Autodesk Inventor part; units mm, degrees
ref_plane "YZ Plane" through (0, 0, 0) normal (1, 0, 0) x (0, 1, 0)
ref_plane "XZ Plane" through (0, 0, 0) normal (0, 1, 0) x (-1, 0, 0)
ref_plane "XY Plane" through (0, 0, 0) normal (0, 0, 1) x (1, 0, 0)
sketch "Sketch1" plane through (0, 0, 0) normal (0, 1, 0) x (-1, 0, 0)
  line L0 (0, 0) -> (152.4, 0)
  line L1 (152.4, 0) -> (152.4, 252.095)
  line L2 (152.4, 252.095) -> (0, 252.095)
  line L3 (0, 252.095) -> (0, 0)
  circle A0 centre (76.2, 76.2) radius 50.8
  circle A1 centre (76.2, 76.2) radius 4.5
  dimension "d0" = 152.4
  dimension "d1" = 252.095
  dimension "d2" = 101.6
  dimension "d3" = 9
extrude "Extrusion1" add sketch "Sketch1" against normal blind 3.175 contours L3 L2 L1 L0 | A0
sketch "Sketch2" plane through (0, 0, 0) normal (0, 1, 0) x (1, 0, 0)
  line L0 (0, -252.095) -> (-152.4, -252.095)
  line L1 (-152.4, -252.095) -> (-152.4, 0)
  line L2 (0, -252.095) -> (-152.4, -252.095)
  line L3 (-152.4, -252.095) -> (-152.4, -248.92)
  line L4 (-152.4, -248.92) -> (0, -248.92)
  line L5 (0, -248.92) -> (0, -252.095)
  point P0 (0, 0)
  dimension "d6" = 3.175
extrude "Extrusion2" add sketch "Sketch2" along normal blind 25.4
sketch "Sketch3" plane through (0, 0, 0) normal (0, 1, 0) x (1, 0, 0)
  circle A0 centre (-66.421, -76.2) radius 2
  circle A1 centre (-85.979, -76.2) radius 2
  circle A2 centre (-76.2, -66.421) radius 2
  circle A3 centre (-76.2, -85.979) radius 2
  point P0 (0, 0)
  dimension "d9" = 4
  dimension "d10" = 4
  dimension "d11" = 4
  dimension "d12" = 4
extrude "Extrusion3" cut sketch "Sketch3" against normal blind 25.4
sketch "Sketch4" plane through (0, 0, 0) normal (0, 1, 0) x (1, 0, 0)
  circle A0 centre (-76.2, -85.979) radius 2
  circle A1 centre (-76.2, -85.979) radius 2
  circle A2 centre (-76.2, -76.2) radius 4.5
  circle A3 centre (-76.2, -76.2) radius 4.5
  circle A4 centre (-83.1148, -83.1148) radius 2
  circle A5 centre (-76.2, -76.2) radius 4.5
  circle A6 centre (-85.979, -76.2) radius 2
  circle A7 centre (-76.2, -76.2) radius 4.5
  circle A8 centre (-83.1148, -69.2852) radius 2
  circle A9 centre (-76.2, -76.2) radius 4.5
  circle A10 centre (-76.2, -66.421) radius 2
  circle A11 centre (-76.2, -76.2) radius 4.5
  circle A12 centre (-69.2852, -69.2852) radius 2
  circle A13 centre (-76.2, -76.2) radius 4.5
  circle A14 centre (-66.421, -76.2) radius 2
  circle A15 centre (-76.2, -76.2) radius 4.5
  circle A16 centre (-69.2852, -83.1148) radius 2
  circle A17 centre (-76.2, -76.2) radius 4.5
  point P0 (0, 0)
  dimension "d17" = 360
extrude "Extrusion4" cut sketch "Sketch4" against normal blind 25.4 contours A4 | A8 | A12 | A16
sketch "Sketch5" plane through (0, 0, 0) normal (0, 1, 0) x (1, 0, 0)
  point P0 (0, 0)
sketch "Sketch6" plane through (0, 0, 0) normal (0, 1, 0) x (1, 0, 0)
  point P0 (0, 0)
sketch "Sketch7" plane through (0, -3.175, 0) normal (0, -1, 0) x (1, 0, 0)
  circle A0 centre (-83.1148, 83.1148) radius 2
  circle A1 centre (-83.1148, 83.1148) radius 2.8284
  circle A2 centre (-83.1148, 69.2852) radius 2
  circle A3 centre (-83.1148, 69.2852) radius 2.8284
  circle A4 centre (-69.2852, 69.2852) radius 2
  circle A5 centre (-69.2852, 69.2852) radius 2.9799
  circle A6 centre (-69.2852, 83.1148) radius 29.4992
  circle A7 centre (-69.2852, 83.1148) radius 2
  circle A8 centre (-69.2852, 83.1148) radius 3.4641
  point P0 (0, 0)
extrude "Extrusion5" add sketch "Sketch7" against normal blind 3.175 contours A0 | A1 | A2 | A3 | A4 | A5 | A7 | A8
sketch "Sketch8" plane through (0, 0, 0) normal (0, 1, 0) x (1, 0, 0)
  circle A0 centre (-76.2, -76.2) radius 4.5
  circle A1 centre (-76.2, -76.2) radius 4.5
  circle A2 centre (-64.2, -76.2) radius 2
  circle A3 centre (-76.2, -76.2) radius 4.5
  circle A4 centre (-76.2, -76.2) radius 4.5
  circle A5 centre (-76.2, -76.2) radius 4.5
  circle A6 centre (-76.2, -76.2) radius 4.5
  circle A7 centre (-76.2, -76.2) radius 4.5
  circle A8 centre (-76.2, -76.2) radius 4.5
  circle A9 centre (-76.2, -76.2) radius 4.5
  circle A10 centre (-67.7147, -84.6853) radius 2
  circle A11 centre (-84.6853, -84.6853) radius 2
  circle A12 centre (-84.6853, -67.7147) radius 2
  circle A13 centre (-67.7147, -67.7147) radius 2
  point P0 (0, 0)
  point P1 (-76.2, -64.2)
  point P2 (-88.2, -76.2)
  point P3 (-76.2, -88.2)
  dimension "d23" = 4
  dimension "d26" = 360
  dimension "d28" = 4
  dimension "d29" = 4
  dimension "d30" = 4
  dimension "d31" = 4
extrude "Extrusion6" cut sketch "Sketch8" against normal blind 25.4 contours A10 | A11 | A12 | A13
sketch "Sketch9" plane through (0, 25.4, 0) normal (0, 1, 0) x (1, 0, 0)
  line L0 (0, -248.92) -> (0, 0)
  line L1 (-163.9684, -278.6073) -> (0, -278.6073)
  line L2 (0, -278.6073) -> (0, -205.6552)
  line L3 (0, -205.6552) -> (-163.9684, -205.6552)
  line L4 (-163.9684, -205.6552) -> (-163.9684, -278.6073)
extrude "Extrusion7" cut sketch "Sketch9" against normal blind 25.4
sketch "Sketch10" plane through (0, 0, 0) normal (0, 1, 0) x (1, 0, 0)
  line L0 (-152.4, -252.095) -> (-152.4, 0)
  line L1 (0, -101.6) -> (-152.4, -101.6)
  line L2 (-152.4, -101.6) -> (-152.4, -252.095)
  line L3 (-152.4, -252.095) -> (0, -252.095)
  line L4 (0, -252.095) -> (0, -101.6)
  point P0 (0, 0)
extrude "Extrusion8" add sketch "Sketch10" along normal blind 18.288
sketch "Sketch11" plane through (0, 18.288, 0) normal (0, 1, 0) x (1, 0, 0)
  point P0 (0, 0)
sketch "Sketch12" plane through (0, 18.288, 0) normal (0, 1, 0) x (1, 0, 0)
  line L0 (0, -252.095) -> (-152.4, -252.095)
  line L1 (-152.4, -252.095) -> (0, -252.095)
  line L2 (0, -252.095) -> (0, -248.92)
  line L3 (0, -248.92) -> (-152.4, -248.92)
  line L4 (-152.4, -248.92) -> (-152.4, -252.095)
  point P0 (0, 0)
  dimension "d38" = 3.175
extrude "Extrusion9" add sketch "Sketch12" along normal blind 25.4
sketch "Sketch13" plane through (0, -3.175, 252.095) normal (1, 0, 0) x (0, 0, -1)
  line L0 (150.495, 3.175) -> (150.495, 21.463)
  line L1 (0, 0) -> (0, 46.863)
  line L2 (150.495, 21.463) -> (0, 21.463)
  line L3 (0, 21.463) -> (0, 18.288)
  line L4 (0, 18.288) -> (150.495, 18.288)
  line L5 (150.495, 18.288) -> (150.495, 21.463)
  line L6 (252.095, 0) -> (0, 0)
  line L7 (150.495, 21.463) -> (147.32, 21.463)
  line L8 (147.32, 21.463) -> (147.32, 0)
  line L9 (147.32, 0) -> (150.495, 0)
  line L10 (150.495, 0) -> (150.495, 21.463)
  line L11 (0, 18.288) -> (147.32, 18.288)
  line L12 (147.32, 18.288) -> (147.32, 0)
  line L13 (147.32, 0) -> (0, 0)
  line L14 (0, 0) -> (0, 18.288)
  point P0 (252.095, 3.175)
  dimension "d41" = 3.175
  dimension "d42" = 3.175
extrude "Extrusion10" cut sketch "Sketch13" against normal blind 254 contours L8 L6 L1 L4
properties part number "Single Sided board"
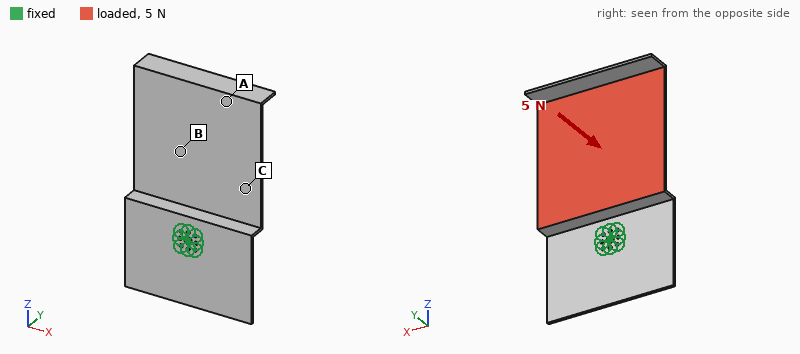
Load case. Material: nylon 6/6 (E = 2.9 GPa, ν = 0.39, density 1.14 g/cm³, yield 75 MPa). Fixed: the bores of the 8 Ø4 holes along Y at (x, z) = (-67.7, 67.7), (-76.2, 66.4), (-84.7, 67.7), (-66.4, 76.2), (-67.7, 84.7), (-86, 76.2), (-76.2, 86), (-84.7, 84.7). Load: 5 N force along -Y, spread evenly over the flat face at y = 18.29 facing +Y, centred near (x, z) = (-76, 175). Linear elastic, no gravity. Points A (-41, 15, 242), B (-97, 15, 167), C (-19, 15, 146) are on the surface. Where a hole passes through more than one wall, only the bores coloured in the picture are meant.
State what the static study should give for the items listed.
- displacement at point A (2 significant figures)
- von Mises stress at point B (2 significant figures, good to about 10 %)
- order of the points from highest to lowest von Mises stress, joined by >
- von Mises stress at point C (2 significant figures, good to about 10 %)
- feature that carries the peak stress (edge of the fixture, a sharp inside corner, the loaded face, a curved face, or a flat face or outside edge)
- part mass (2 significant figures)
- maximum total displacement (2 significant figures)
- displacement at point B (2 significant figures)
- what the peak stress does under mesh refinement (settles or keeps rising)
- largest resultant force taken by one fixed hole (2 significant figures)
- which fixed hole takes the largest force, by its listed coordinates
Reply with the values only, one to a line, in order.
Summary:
3.1 mm
0.39 MPa
C > B > A
0.66 MPa
edge of the fixture
160 g
3.4 mm
1.3 mm
keeps rising
7.1 N
(-76.2, 86)
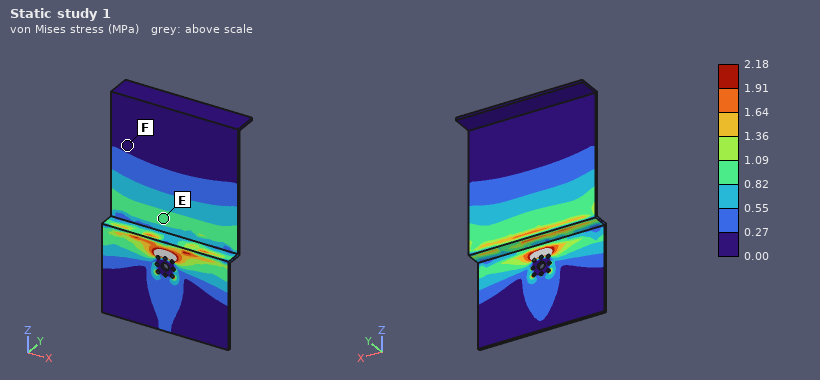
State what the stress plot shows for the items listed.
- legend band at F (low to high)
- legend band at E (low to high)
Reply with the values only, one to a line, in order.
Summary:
0.00 to 0.27 MPa
0.82 to 1.09 MPa
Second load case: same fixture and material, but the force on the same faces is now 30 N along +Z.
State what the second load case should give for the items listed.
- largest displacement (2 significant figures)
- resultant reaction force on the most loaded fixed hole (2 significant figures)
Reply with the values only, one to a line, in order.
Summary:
2.7 mm
8.2 N
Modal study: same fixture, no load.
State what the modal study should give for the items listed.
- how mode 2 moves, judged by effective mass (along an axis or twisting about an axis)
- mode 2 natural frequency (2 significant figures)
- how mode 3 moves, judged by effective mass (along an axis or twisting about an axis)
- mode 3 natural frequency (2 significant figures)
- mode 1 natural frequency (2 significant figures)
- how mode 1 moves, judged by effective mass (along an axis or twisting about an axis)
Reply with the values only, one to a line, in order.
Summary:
twisting about Z
56 Hz
along X
110 Hz
21 Hz
along Y
